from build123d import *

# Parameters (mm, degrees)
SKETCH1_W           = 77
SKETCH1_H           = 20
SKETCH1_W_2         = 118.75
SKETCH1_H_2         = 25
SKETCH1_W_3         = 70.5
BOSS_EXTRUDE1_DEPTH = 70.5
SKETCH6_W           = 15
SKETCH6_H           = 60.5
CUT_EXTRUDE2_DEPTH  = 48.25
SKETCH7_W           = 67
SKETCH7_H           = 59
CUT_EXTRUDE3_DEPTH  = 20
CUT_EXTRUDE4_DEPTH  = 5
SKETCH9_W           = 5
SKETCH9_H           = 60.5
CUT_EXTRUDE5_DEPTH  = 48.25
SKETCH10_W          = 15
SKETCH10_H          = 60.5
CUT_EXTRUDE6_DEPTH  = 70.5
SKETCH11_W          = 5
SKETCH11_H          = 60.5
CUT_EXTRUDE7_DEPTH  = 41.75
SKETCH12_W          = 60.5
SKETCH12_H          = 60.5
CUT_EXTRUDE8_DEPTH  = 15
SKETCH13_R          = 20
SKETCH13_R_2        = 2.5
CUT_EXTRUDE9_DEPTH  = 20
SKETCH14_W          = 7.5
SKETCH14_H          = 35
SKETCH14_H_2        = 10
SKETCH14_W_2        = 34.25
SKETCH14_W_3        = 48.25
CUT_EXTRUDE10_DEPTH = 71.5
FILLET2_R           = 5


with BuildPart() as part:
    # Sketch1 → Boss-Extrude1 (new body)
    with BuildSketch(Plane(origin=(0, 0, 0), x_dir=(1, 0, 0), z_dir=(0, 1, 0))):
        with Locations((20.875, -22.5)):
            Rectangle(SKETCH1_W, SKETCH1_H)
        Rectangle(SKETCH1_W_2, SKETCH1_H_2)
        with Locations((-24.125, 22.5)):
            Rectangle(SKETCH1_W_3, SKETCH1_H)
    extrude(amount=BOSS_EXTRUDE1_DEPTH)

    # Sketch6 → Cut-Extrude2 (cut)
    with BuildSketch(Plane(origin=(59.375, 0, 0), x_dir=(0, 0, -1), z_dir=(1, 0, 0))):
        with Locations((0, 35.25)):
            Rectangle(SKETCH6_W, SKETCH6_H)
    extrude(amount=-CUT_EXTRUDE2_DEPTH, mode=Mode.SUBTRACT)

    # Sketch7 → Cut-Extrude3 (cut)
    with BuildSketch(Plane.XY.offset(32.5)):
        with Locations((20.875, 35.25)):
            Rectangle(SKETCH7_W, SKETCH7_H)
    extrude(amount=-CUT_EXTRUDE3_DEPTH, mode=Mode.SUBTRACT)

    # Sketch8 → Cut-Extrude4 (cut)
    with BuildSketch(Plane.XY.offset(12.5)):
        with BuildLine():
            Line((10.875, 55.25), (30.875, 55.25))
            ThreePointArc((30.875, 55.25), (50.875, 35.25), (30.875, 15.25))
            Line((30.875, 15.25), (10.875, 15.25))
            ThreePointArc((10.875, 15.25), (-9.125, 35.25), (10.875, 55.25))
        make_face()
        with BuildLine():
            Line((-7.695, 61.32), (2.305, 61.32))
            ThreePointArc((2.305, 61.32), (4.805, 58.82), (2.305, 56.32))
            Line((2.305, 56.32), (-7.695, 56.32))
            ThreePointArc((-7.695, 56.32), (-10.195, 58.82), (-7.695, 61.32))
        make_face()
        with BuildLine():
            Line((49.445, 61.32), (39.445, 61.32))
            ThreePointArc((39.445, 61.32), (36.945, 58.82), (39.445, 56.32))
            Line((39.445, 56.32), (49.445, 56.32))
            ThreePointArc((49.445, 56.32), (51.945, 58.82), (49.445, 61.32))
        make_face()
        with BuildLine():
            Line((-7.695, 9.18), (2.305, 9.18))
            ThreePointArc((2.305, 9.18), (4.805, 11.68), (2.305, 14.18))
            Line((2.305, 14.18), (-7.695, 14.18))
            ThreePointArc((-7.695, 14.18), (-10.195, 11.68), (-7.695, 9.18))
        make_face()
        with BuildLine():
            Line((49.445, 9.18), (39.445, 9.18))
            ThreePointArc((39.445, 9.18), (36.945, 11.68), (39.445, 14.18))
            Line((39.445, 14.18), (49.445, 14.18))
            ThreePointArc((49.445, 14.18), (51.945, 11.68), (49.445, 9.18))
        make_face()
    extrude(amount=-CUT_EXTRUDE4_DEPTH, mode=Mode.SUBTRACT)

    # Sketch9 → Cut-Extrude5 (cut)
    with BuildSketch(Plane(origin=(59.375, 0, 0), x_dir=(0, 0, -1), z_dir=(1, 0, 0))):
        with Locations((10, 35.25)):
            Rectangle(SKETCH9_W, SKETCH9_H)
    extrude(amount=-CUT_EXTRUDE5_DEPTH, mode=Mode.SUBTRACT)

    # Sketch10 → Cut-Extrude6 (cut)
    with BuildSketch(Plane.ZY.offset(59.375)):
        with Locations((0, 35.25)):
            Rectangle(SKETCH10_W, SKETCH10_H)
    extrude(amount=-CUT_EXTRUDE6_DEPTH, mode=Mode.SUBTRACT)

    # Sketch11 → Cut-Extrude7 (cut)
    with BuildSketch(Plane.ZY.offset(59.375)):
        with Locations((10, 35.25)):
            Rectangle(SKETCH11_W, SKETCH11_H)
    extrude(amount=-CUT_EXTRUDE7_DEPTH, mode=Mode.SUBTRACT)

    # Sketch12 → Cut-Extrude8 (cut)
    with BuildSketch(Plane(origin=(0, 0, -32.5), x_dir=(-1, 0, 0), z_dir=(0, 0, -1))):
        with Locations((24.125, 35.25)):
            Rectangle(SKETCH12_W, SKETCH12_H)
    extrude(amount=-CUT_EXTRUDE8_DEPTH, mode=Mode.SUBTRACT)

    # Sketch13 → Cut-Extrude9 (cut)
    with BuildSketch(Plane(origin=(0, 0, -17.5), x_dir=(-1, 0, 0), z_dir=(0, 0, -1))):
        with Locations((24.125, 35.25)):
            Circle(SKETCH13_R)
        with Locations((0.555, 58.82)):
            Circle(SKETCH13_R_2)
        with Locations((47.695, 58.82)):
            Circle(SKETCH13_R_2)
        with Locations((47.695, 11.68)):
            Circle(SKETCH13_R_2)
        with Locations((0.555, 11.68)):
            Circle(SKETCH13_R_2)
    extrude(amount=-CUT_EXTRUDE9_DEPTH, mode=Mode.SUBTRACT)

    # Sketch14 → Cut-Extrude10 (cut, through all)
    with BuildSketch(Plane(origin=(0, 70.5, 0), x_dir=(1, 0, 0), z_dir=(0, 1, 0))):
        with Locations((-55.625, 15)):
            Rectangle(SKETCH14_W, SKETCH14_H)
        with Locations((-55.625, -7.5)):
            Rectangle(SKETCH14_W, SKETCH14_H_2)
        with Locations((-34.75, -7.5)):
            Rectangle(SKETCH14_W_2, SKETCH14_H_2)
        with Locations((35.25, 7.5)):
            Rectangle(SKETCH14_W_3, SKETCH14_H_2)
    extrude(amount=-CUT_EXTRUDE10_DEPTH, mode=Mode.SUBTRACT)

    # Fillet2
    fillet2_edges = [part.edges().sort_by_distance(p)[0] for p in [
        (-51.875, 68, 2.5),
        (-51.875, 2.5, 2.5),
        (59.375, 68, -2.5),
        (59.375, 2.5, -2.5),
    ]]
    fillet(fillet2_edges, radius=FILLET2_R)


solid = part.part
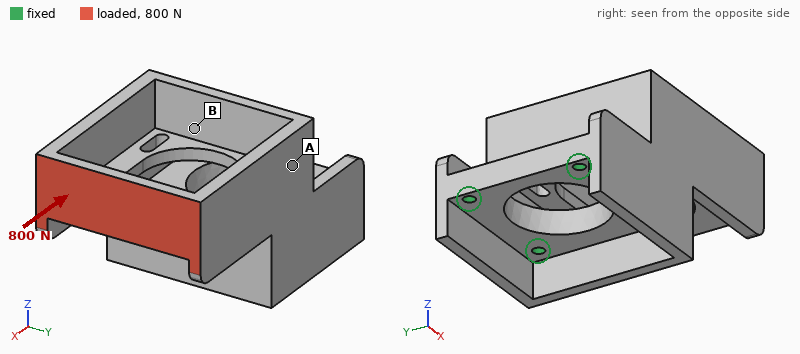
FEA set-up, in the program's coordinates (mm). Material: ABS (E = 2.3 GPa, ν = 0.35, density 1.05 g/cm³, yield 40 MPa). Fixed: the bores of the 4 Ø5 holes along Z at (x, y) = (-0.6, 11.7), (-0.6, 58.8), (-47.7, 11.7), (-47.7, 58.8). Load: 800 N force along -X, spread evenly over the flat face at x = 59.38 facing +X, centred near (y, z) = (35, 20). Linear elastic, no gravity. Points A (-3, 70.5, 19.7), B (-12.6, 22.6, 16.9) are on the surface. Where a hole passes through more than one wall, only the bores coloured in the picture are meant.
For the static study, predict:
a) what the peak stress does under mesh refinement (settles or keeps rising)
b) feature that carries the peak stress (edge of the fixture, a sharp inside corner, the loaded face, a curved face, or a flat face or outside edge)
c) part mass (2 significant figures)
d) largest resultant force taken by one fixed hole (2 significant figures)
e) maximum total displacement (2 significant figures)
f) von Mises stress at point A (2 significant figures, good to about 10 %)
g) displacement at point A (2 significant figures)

keeps rising
edge of the fixture
110 g
330 N
1.5 mm
4.1 MPa
0.29 mm
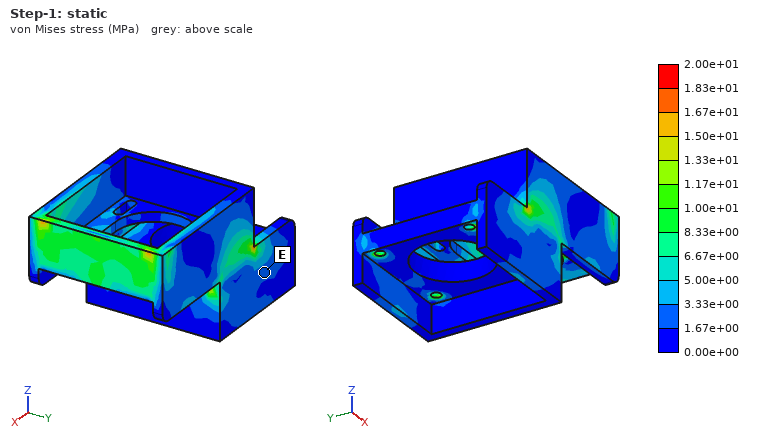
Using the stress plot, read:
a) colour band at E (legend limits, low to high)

1.67e+00 to 3.33e+00 MPa
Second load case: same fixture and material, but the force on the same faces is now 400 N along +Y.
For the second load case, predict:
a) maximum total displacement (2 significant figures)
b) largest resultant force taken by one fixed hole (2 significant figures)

1.4 mm
360 N
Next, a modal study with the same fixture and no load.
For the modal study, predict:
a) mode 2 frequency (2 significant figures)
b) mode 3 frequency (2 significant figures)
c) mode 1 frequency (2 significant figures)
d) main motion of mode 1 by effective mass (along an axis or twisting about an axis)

640 Hz
890 Hz
560 Hz
along Y
